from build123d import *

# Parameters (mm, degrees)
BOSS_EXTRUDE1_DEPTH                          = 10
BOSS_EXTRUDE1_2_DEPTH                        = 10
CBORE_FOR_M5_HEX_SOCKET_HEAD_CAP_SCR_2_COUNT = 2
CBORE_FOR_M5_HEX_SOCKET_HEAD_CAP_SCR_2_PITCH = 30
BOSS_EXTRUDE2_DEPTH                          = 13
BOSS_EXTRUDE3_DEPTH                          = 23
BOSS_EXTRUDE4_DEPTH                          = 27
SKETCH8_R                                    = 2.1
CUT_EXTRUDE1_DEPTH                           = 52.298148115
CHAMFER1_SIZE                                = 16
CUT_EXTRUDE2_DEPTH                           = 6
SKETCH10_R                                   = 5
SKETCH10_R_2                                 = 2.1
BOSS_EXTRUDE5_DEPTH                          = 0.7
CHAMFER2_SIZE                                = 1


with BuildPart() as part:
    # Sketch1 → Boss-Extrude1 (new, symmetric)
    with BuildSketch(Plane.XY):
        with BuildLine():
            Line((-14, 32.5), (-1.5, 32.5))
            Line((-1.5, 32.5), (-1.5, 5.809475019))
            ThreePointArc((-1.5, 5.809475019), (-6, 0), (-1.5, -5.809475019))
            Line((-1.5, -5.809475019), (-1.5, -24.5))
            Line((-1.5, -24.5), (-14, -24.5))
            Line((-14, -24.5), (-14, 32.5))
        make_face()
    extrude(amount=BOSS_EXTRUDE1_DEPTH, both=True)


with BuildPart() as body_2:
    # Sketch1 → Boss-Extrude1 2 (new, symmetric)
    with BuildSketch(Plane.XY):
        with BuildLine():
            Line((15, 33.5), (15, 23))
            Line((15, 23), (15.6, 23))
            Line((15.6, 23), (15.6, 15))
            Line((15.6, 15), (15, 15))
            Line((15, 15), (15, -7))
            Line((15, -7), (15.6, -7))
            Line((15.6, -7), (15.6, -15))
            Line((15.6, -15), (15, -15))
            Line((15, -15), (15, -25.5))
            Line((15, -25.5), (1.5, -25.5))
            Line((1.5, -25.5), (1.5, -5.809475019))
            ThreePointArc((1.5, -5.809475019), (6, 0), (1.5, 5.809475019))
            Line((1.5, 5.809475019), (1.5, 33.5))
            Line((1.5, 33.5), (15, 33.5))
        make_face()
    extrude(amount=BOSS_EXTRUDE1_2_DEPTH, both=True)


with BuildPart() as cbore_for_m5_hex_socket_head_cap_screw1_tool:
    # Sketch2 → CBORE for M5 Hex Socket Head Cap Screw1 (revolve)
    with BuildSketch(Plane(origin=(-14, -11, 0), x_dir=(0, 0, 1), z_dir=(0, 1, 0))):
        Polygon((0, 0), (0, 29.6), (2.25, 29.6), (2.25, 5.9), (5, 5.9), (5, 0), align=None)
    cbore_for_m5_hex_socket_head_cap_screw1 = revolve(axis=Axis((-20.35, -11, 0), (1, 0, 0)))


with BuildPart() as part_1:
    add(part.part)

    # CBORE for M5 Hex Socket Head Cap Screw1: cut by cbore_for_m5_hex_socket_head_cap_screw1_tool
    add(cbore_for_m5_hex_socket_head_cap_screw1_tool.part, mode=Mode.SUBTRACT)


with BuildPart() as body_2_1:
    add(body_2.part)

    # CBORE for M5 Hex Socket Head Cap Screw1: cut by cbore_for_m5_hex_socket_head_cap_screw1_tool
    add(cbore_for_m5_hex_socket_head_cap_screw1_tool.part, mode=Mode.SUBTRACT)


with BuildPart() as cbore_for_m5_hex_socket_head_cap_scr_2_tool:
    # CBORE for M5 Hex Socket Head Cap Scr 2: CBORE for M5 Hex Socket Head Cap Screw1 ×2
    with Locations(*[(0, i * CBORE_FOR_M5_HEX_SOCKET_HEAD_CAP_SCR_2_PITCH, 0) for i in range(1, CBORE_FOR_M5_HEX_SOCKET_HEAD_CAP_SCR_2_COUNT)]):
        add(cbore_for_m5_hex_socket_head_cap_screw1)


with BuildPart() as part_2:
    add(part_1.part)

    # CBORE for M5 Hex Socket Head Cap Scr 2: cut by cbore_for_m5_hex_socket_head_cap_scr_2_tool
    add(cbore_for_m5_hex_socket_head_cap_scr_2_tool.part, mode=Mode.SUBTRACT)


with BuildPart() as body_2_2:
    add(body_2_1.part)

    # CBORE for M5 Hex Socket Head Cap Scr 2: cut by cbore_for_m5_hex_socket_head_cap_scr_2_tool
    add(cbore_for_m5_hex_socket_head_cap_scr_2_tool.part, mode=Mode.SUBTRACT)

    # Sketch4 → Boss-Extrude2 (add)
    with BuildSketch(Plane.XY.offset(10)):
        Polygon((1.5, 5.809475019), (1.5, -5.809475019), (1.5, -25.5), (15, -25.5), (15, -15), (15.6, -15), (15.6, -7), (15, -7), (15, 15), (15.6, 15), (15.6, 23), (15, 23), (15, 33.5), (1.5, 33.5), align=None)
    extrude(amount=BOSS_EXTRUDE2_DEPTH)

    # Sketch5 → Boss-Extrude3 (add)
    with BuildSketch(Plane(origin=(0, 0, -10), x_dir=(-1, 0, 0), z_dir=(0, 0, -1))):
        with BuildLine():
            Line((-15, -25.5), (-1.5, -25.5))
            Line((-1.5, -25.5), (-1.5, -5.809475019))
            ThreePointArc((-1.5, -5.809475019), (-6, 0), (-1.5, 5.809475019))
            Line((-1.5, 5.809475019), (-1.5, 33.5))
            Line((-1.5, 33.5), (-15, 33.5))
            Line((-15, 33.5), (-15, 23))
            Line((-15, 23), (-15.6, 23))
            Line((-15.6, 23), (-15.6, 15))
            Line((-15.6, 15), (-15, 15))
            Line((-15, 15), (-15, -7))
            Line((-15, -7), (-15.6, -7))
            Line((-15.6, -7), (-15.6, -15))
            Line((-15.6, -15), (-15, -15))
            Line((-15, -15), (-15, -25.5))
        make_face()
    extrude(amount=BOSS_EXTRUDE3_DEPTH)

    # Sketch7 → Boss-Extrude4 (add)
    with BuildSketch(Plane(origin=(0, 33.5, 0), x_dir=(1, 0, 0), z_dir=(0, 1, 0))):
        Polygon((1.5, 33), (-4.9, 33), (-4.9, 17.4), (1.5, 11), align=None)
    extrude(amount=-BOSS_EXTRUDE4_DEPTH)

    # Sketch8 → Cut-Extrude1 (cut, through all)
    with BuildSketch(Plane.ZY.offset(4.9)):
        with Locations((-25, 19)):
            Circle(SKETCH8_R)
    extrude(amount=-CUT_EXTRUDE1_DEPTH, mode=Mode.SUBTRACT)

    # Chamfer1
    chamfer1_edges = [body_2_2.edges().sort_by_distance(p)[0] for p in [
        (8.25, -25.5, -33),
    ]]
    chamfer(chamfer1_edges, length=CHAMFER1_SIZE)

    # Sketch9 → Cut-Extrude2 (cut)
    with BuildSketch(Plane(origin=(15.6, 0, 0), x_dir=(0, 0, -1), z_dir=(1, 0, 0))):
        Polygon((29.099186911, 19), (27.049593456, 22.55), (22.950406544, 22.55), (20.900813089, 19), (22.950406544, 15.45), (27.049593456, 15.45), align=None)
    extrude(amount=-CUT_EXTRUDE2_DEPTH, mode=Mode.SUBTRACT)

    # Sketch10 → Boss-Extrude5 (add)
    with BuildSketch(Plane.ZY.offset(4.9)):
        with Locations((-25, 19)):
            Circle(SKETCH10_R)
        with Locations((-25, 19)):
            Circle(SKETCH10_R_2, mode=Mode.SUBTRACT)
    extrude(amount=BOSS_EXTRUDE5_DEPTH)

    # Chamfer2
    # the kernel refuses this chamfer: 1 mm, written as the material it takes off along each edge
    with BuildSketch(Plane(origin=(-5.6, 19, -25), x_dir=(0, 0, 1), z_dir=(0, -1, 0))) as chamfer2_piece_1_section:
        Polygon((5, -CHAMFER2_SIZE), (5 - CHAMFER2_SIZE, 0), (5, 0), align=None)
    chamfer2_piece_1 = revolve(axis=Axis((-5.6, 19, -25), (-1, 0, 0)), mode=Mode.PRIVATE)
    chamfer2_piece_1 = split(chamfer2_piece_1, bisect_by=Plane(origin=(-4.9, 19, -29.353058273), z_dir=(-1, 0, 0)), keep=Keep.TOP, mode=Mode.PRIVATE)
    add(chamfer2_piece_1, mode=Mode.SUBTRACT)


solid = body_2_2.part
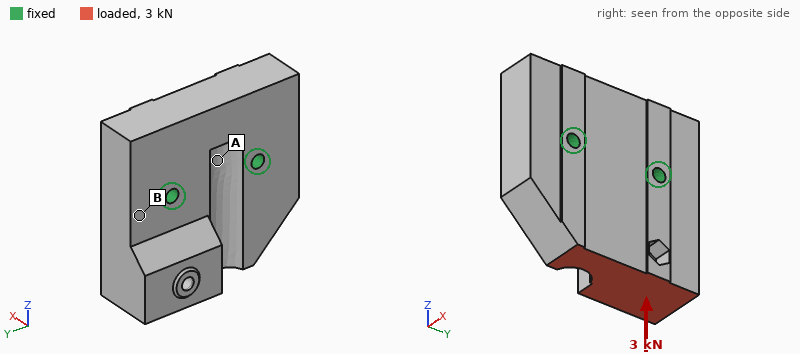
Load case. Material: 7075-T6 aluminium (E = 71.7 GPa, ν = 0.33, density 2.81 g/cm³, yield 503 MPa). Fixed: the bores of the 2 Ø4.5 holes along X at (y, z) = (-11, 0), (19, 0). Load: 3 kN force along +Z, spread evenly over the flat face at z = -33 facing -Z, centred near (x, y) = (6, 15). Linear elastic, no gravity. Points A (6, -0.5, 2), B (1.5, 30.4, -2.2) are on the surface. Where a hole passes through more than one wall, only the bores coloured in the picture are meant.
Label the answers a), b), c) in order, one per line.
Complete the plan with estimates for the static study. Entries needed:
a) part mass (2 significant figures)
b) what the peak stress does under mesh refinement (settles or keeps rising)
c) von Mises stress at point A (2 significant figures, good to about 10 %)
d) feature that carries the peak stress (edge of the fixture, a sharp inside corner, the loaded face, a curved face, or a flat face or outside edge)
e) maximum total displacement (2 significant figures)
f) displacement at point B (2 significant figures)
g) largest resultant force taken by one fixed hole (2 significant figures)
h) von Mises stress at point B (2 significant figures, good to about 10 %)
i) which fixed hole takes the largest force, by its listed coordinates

a) 120 g
b) keeps rising
c) 2.5 MPa
d) edge of the fixture
e) 9.5 µm
f) 2.5 µm
g) 2.5 kN
h) 7.0 MPa
i) (19, 0)
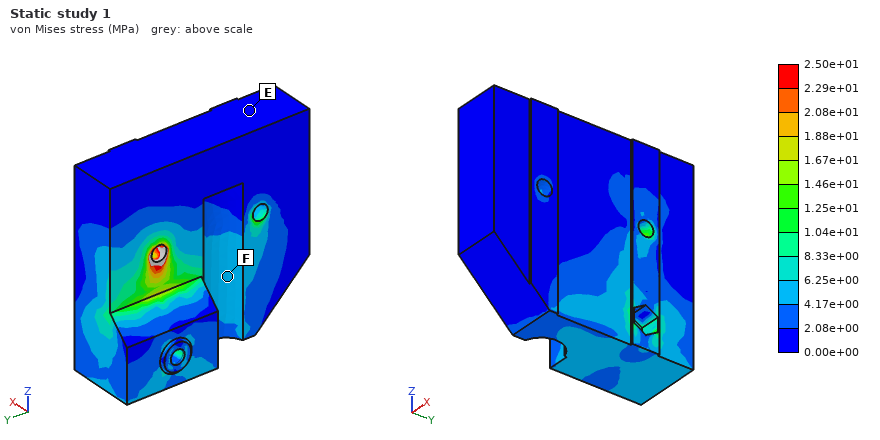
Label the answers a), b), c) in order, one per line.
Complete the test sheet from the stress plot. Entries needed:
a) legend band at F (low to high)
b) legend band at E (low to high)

a) 4.17e+00 to 6.25e+00 MPa
b) 0.00e+00 to 2.08e+00 MPa
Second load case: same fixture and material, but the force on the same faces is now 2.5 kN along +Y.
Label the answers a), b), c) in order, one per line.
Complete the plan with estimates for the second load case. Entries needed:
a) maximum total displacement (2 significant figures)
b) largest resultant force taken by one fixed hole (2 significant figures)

a) 16 µm
b) 2.8 kN
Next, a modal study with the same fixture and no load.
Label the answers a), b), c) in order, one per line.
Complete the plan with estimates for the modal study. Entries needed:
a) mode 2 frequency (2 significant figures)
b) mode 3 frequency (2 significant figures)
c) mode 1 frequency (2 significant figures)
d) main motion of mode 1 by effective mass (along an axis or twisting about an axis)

a) 12 kHz
b) 14 kHz
c) 7300 Hz
d) along X
